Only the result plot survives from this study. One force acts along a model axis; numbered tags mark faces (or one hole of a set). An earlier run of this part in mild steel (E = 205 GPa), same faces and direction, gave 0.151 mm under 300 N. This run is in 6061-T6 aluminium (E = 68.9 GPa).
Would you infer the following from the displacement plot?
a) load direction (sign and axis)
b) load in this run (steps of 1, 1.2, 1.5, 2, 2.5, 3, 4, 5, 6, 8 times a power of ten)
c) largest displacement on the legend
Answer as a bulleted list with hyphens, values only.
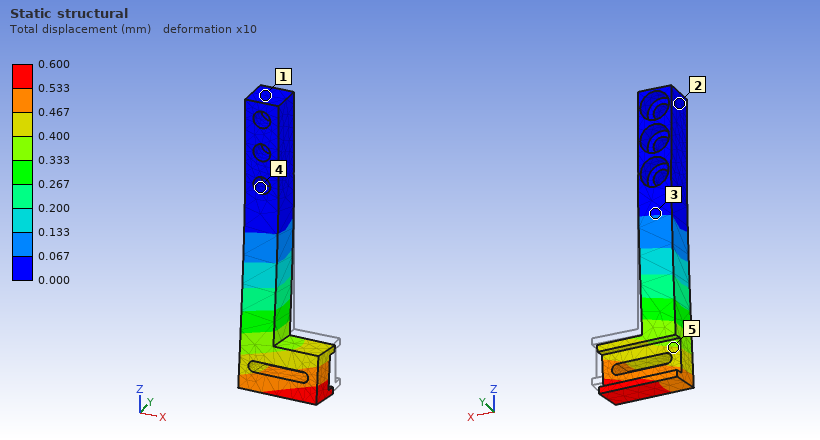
- -Y
- 400 N
- 0.600 mm
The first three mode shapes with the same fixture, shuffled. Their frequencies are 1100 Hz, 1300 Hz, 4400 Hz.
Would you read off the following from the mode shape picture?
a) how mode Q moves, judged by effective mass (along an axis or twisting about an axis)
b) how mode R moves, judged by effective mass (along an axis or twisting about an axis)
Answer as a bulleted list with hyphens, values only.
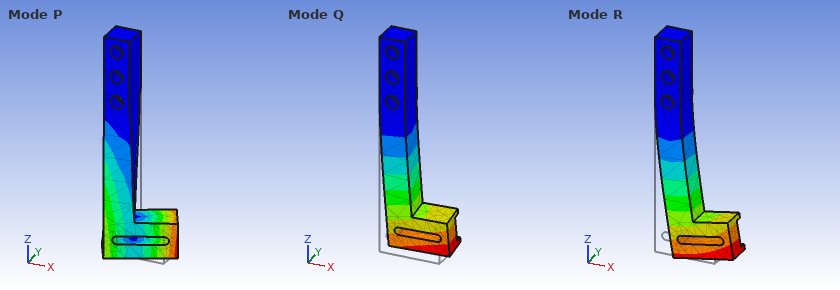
- along Y
- along X
